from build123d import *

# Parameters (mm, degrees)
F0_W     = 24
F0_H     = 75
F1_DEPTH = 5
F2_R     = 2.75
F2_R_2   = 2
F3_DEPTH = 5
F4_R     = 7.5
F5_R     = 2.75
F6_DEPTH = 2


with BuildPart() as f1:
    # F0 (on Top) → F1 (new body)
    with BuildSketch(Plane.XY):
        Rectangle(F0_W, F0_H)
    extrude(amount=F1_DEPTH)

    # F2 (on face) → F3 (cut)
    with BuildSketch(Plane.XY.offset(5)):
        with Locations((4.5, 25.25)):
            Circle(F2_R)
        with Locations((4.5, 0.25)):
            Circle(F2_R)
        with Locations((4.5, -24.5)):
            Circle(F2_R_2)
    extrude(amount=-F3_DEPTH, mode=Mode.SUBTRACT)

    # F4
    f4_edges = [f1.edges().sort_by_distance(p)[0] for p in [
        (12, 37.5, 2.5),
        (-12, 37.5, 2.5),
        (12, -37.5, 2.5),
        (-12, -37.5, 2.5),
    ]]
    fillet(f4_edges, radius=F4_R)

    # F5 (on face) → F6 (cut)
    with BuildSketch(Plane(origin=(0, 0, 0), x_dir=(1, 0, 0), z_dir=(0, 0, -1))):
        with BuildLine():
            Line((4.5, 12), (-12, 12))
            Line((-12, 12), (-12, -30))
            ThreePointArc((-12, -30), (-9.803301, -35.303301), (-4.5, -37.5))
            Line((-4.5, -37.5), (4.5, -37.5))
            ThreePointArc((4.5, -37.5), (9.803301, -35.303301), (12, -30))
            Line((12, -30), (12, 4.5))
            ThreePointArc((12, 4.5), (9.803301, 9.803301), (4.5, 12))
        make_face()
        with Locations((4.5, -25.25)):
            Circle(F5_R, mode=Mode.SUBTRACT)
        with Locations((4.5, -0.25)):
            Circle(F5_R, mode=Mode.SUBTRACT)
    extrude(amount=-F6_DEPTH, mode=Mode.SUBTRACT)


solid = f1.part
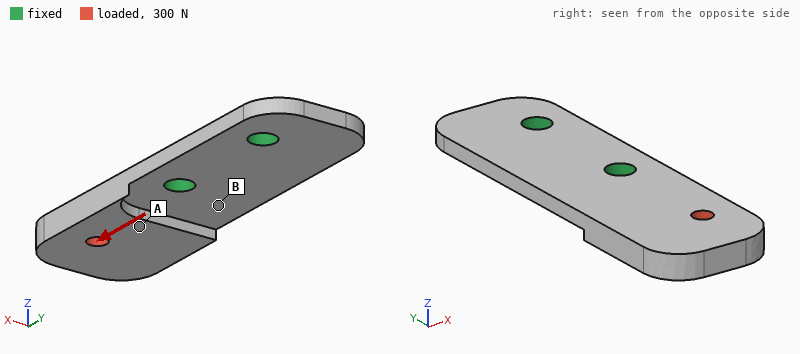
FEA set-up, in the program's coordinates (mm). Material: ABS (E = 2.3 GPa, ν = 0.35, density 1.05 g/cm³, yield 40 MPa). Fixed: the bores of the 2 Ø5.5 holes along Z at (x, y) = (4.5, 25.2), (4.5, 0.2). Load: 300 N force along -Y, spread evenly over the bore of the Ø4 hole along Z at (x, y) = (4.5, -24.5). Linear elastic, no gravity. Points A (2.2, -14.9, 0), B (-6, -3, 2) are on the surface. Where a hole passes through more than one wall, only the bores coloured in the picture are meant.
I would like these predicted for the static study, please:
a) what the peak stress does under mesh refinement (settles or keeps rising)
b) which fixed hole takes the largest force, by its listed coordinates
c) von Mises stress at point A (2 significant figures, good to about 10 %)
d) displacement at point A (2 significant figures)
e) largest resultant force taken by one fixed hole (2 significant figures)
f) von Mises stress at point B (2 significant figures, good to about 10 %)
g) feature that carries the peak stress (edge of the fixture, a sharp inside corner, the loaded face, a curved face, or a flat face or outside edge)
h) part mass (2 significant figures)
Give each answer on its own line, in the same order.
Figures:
keeps rising
(4.5, 0.2)
2.5 MPa
0.26 mm
270 N
6.0 MPa
a sharp inside corner
6.6 g
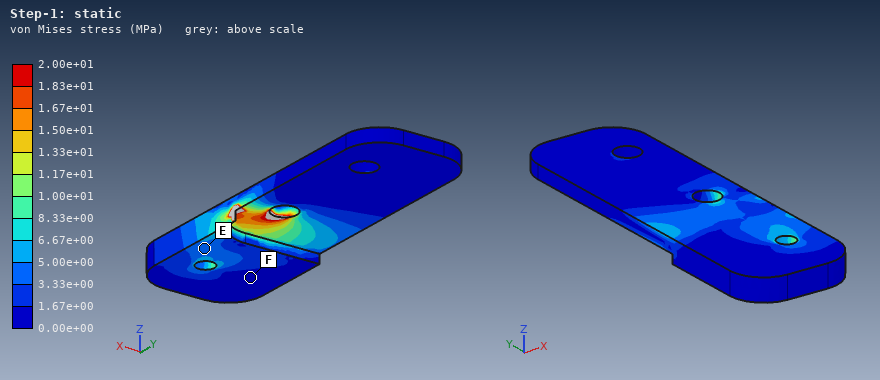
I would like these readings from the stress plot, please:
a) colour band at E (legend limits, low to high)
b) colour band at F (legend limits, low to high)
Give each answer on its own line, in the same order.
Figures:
3.33e+00 to 5.00e+00 MPa
0.00e+00 to 1.67e+00 MPa
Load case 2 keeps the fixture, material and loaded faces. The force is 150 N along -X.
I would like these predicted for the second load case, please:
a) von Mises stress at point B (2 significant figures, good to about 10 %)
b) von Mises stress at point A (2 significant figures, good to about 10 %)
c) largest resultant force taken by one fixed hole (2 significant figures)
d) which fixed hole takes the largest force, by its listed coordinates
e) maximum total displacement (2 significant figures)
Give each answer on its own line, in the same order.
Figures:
6.1 MPa
2.3 MPa
260 N
(4.5, 0.2)
0.39 mm
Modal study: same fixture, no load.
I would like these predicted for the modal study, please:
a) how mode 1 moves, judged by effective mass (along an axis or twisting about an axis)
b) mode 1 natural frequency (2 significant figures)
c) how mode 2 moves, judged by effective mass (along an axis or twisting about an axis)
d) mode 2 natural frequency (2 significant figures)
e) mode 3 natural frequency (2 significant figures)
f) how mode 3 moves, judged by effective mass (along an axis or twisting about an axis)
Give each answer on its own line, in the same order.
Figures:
along Z
470 Hz
twisting about Y
1600 Hz
2100 Hz
along X
